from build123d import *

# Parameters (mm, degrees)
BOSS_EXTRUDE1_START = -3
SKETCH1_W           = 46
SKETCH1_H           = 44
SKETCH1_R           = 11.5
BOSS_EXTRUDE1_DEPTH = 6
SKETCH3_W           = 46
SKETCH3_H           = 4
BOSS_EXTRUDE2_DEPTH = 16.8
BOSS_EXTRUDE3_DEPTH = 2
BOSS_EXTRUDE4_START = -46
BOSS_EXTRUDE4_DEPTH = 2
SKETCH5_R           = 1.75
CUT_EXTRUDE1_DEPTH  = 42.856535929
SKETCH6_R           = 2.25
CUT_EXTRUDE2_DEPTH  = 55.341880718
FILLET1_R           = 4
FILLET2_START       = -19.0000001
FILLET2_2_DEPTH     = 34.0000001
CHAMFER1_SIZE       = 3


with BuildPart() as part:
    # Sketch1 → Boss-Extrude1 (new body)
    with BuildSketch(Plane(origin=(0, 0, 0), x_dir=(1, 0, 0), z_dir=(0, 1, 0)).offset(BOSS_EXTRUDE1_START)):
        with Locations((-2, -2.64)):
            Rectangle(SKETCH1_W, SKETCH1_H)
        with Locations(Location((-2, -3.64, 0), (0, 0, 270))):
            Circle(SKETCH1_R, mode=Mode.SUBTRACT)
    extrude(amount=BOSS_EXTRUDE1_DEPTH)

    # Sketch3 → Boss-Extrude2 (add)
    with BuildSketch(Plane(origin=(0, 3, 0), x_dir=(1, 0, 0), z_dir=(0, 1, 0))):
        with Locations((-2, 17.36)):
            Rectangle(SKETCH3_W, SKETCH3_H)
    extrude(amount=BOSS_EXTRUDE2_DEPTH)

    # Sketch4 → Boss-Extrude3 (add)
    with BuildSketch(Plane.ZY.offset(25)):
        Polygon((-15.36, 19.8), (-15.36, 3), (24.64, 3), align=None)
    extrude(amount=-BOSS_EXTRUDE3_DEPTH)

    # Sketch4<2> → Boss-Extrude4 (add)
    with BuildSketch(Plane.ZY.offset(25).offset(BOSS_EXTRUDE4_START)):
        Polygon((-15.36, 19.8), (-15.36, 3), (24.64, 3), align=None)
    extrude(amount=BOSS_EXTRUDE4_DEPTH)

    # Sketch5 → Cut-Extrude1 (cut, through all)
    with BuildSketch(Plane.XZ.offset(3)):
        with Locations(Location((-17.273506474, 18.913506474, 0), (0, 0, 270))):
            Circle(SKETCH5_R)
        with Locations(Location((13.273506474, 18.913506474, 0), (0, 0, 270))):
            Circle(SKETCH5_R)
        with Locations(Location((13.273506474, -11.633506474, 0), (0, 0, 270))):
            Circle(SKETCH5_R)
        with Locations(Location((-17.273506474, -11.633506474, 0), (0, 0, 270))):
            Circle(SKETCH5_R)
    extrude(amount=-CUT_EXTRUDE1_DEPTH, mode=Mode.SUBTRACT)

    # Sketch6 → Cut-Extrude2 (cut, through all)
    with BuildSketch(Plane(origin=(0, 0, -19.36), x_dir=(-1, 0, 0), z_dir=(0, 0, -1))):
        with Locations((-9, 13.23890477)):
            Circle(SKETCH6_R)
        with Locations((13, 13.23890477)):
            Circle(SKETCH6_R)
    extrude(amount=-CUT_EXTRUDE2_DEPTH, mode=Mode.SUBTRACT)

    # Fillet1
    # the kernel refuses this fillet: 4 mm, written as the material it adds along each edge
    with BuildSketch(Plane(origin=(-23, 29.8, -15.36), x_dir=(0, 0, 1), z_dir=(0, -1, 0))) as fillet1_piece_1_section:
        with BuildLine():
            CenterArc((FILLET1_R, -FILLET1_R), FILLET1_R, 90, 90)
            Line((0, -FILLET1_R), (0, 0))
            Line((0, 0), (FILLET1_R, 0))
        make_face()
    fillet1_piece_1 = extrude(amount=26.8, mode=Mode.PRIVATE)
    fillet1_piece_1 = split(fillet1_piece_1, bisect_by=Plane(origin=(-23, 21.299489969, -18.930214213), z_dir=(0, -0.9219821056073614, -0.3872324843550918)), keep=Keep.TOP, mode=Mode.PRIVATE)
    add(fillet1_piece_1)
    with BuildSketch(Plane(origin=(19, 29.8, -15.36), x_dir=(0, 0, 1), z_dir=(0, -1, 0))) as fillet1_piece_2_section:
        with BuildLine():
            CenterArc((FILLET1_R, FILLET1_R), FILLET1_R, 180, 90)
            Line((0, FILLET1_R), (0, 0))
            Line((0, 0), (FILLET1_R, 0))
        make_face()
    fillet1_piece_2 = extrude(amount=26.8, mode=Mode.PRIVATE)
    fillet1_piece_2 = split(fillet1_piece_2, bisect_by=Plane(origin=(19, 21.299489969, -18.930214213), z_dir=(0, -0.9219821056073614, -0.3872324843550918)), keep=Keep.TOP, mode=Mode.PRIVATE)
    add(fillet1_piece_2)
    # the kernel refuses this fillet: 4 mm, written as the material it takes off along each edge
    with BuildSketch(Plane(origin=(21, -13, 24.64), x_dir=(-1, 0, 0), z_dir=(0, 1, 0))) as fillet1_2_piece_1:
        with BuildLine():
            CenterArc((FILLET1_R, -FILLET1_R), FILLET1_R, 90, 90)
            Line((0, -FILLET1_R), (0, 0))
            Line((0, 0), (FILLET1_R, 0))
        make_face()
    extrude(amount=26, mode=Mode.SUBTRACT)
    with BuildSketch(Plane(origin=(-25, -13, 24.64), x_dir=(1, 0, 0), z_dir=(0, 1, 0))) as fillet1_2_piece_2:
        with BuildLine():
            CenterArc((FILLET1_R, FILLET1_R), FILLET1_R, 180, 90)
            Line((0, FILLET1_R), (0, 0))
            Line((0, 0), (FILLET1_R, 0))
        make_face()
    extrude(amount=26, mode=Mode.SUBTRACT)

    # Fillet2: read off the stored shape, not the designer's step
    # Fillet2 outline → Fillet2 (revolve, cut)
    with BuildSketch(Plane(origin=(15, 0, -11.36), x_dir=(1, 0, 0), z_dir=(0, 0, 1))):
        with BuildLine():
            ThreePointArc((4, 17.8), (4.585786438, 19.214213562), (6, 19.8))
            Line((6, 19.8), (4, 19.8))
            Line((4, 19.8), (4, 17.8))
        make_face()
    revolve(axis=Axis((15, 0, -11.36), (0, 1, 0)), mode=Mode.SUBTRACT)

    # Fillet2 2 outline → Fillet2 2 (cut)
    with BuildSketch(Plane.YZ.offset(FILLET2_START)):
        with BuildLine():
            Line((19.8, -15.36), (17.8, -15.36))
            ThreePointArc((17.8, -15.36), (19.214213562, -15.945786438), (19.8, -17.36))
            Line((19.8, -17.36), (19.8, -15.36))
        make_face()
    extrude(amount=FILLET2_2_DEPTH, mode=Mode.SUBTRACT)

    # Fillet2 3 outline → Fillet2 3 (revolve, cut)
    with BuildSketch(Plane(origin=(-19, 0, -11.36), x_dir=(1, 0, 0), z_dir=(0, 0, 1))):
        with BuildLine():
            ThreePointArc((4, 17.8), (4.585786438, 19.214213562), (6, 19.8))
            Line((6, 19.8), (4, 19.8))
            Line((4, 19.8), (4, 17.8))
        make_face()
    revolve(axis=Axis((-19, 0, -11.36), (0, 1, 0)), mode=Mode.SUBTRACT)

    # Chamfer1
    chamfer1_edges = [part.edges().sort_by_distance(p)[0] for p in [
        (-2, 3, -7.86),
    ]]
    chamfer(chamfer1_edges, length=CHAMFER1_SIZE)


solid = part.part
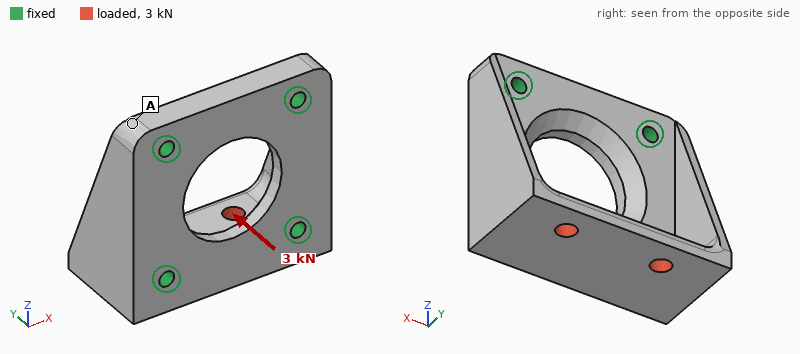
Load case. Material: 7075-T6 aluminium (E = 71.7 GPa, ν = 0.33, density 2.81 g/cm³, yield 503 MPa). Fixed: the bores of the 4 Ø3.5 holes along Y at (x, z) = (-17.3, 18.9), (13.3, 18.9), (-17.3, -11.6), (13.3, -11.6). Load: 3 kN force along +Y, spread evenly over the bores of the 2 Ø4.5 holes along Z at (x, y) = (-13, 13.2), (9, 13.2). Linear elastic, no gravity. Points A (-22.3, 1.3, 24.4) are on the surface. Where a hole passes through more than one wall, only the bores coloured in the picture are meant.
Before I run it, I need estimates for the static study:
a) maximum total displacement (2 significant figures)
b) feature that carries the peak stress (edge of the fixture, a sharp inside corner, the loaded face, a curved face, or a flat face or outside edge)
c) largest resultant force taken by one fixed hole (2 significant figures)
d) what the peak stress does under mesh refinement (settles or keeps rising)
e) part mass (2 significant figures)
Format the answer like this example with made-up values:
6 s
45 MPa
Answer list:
26 µm
edge of the fixture
1.6 kN
keeps rising
38 g
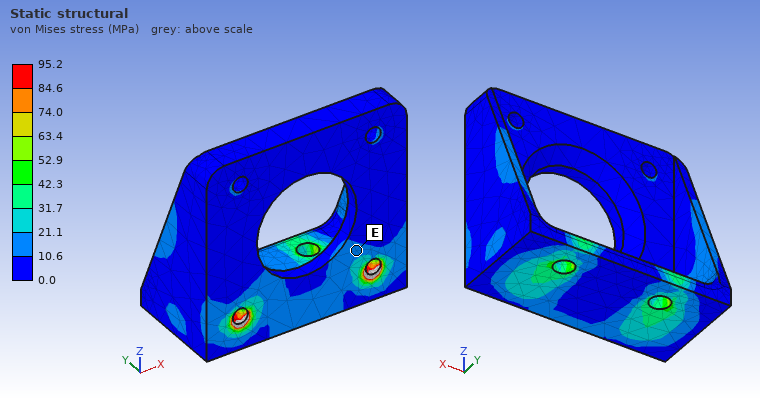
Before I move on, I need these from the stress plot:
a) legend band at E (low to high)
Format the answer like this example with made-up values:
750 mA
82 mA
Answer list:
10.6 to 21.1 MPa
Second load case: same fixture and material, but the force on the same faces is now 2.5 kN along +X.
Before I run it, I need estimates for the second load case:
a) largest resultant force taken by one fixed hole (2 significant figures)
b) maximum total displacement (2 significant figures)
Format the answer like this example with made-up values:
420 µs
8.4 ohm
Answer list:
1.6 kN
21 µm
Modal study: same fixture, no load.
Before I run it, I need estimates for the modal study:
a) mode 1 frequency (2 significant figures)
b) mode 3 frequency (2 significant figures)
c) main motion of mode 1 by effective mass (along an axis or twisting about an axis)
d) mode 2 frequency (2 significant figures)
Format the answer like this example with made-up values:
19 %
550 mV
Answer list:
11 kHz
18 kHz
along Z
18 kHz
